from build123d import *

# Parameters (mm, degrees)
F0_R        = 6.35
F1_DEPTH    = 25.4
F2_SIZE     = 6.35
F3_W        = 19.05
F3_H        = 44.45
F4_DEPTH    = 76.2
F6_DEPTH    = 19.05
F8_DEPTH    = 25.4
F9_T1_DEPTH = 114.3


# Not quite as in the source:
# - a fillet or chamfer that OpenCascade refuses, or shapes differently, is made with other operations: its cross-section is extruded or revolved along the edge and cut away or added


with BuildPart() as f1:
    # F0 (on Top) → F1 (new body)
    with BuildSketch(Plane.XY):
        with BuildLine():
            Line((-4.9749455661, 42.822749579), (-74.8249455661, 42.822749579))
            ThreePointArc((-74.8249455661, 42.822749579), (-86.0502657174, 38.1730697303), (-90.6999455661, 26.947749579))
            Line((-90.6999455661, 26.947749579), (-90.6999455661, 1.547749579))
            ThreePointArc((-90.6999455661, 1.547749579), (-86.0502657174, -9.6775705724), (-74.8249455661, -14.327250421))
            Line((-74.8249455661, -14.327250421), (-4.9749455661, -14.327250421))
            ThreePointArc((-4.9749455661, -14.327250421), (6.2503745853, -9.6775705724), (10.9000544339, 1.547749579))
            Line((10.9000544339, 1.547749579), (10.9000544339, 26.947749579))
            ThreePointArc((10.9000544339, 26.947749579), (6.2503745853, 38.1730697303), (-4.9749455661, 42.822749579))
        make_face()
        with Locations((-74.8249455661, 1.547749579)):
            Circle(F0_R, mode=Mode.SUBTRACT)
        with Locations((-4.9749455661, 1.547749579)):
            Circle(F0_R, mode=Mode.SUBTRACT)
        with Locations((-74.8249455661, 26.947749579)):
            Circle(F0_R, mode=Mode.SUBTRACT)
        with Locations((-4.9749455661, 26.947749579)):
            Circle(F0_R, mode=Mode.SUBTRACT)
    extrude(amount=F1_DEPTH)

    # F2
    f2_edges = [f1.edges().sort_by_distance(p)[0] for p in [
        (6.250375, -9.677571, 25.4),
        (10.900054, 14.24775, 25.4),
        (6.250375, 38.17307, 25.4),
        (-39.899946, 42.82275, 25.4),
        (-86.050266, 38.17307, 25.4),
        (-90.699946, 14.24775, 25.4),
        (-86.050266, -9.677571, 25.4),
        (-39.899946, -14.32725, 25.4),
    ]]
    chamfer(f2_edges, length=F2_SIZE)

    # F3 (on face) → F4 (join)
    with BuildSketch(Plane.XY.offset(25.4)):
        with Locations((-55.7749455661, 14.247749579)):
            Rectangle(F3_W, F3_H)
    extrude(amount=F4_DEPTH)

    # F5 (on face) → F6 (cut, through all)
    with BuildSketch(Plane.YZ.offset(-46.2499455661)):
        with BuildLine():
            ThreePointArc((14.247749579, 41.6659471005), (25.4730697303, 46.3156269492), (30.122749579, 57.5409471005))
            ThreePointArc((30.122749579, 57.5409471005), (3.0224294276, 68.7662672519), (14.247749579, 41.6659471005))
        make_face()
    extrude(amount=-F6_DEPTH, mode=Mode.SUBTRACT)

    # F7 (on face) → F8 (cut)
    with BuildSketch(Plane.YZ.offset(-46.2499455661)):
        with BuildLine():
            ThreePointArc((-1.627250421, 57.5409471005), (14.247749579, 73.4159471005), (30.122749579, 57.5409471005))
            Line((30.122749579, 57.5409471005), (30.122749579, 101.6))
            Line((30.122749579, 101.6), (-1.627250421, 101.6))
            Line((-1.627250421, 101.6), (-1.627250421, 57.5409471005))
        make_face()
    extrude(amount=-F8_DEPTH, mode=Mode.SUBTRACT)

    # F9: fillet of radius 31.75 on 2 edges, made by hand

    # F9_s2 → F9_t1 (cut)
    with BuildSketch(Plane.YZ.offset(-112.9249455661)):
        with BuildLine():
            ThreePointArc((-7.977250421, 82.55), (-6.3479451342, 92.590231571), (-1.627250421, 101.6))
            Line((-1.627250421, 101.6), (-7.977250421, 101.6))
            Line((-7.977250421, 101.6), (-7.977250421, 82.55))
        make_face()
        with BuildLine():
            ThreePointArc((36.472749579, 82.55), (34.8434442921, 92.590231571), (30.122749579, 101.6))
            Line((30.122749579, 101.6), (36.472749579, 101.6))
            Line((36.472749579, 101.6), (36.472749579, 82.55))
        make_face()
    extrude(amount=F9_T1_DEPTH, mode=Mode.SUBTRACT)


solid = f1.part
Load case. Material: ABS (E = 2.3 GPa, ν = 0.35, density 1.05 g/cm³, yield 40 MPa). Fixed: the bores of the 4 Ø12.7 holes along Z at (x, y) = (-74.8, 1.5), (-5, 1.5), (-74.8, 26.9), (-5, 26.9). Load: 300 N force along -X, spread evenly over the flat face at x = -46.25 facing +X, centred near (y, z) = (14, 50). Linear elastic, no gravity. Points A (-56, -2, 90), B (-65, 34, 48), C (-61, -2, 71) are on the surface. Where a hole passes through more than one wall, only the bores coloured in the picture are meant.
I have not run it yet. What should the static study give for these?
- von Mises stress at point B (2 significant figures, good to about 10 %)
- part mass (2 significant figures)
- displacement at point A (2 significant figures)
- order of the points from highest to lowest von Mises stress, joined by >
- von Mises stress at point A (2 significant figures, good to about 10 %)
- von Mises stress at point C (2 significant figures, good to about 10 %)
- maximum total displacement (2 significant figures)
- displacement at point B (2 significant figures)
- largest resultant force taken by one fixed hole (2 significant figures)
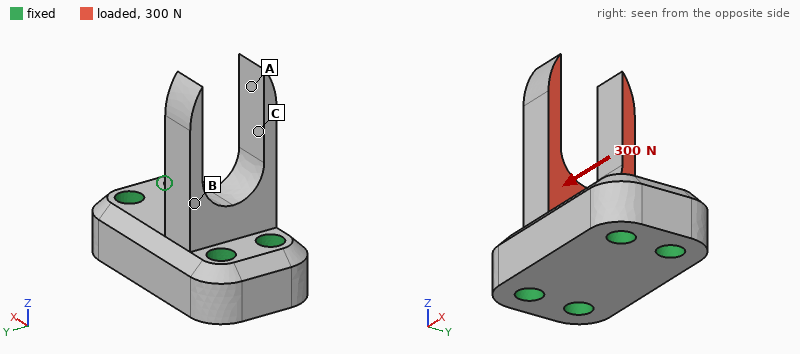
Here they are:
2.9 MPa
160 g
0.30 mm
B > C > A
0.25 MPa
0.83 MPa
0.38 mm
0.067 mm
150 N
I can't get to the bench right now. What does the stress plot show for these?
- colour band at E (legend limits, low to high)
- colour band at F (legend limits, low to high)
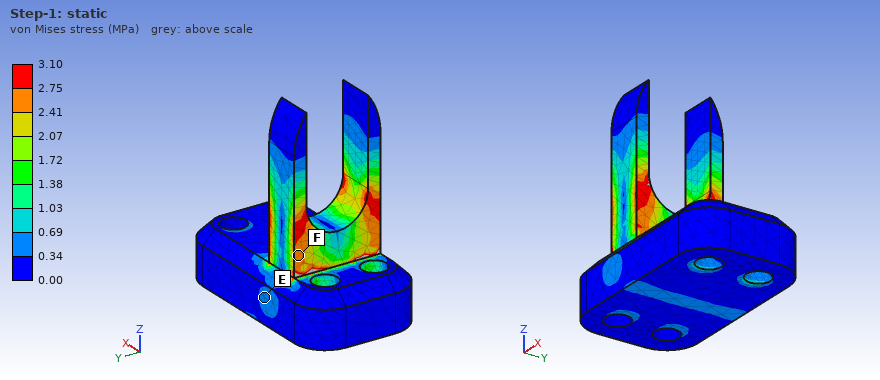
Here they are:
0.34 to 0.69 MPa
2.41 to 2.75 MPa
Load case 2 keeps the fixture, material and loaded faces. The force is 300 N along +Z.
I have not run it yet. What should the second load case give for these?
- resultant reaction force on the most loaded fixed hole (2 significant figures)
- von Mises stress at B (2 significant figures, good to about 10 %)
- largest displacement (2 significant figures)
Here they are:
96 N
0.72 MPa
0.17 mm
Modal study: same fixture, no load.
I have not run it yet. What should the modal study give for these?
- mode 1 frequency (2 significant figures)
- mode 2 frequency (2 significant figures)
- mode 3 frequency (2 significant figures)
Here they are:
630 Hz
640 Hz
1100 Hz
